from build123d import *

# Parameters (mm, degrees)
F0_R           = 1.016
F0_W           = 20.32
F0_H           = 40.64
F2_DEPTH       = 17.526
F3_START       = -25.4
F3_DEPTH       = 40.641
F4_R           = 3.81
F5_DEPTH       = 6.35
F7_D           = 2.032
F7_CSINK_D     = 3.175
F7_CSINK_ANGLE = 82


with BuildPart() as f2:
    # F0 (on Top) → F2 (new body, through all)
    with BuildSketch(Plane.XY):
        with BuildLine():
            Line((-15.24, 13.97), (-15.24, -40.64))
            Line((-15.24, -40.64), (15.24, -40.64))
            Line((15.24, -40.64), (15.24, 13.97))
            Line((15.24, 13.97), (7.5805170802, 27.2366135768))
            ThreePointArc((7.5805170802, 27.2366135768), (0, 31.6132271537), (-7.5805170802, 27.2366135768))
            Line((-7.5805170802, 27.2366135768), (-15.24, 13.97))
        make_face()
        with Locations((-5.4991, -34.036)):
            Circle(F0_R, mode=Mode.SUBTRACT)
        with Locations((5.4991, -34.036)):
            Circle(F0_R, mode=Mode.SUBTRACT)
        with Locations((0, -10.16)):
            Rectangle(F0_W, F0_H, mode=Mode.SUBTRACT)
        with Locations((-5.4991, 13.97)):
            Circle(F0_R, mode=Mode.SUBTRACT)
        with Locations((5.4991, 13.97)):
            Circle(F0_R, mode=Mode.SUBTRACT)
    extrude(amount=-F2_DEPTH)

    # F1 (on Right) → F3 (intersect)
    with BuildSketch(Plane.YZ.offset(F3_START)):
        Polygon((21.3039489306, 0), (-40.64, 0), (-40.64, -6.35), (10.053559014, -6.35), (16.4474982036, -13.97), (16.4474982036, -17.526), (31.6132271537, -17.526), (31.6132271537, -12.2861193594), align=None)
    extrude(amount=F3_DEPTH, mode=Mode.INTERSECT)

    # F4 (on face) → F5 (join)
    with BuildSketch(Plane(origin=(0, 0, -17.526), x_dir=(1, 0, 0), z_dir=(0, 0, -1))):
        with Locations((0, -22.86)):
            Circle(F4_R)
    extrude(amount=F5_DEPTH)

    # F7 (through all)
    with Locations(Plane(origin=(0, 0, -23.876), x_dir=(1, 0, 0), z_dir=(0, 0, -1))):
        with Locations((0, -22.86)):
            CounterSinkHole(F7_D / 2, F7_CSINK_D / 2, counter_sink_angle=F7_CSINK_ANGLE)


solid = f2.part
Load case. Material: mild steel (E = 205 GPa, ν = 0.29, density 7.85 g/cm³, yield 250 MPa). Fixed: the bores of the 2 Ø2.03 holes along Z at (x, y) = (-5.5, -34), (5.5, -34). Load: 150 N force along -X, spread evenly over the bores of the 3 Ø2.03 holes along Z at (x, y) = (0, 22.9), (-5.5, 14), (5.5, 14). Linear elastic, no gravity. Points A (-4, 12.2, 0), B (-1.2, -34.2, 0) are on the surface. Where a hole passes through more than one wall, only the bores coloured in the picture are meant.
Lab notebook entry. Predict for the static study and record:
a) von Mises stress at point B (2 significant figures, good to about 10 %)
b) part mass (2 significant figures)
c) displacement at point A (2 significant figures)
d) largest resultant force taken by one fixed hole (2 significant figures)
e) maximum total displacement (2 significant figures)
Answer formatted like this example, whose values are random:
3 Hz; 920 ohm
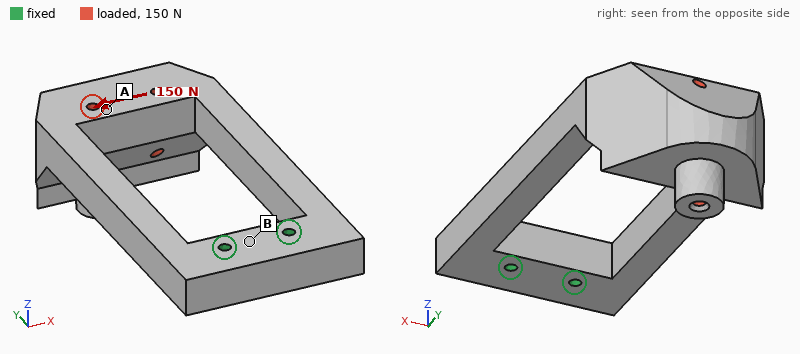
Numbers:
11 MPa; 84 g; 54 µm; 560 N; 75 µm
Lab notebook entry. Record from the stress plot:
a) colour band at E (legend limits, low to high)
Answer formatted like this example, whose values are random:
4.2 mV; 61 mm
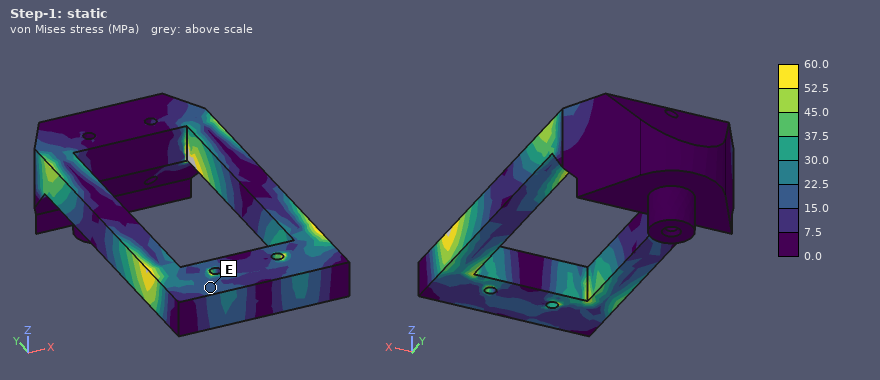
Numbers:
15.0 to 22.5 MPa
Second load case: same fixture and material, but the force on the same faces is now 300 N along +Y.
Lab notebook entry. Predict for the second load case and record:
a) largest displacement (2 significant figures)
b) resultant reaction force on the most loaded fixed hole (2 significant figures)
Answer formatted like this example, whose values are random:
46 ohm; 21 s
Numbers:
91 µm; 170 N
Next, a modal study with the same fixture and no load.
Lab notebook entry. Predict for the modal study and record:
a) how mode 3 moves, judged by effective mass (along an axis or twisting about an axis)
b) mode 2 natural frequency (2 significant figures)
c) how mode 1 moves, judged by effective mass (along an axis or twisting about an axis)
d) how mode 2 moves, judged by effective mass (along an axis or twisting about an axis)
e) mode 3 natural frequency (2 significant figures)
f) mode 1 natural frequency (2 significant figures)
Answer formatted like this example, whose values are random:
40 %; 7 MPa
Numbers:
twisting about Y; 1100 Hz; along Z; along X; 2400 Hz; 590 Hz
